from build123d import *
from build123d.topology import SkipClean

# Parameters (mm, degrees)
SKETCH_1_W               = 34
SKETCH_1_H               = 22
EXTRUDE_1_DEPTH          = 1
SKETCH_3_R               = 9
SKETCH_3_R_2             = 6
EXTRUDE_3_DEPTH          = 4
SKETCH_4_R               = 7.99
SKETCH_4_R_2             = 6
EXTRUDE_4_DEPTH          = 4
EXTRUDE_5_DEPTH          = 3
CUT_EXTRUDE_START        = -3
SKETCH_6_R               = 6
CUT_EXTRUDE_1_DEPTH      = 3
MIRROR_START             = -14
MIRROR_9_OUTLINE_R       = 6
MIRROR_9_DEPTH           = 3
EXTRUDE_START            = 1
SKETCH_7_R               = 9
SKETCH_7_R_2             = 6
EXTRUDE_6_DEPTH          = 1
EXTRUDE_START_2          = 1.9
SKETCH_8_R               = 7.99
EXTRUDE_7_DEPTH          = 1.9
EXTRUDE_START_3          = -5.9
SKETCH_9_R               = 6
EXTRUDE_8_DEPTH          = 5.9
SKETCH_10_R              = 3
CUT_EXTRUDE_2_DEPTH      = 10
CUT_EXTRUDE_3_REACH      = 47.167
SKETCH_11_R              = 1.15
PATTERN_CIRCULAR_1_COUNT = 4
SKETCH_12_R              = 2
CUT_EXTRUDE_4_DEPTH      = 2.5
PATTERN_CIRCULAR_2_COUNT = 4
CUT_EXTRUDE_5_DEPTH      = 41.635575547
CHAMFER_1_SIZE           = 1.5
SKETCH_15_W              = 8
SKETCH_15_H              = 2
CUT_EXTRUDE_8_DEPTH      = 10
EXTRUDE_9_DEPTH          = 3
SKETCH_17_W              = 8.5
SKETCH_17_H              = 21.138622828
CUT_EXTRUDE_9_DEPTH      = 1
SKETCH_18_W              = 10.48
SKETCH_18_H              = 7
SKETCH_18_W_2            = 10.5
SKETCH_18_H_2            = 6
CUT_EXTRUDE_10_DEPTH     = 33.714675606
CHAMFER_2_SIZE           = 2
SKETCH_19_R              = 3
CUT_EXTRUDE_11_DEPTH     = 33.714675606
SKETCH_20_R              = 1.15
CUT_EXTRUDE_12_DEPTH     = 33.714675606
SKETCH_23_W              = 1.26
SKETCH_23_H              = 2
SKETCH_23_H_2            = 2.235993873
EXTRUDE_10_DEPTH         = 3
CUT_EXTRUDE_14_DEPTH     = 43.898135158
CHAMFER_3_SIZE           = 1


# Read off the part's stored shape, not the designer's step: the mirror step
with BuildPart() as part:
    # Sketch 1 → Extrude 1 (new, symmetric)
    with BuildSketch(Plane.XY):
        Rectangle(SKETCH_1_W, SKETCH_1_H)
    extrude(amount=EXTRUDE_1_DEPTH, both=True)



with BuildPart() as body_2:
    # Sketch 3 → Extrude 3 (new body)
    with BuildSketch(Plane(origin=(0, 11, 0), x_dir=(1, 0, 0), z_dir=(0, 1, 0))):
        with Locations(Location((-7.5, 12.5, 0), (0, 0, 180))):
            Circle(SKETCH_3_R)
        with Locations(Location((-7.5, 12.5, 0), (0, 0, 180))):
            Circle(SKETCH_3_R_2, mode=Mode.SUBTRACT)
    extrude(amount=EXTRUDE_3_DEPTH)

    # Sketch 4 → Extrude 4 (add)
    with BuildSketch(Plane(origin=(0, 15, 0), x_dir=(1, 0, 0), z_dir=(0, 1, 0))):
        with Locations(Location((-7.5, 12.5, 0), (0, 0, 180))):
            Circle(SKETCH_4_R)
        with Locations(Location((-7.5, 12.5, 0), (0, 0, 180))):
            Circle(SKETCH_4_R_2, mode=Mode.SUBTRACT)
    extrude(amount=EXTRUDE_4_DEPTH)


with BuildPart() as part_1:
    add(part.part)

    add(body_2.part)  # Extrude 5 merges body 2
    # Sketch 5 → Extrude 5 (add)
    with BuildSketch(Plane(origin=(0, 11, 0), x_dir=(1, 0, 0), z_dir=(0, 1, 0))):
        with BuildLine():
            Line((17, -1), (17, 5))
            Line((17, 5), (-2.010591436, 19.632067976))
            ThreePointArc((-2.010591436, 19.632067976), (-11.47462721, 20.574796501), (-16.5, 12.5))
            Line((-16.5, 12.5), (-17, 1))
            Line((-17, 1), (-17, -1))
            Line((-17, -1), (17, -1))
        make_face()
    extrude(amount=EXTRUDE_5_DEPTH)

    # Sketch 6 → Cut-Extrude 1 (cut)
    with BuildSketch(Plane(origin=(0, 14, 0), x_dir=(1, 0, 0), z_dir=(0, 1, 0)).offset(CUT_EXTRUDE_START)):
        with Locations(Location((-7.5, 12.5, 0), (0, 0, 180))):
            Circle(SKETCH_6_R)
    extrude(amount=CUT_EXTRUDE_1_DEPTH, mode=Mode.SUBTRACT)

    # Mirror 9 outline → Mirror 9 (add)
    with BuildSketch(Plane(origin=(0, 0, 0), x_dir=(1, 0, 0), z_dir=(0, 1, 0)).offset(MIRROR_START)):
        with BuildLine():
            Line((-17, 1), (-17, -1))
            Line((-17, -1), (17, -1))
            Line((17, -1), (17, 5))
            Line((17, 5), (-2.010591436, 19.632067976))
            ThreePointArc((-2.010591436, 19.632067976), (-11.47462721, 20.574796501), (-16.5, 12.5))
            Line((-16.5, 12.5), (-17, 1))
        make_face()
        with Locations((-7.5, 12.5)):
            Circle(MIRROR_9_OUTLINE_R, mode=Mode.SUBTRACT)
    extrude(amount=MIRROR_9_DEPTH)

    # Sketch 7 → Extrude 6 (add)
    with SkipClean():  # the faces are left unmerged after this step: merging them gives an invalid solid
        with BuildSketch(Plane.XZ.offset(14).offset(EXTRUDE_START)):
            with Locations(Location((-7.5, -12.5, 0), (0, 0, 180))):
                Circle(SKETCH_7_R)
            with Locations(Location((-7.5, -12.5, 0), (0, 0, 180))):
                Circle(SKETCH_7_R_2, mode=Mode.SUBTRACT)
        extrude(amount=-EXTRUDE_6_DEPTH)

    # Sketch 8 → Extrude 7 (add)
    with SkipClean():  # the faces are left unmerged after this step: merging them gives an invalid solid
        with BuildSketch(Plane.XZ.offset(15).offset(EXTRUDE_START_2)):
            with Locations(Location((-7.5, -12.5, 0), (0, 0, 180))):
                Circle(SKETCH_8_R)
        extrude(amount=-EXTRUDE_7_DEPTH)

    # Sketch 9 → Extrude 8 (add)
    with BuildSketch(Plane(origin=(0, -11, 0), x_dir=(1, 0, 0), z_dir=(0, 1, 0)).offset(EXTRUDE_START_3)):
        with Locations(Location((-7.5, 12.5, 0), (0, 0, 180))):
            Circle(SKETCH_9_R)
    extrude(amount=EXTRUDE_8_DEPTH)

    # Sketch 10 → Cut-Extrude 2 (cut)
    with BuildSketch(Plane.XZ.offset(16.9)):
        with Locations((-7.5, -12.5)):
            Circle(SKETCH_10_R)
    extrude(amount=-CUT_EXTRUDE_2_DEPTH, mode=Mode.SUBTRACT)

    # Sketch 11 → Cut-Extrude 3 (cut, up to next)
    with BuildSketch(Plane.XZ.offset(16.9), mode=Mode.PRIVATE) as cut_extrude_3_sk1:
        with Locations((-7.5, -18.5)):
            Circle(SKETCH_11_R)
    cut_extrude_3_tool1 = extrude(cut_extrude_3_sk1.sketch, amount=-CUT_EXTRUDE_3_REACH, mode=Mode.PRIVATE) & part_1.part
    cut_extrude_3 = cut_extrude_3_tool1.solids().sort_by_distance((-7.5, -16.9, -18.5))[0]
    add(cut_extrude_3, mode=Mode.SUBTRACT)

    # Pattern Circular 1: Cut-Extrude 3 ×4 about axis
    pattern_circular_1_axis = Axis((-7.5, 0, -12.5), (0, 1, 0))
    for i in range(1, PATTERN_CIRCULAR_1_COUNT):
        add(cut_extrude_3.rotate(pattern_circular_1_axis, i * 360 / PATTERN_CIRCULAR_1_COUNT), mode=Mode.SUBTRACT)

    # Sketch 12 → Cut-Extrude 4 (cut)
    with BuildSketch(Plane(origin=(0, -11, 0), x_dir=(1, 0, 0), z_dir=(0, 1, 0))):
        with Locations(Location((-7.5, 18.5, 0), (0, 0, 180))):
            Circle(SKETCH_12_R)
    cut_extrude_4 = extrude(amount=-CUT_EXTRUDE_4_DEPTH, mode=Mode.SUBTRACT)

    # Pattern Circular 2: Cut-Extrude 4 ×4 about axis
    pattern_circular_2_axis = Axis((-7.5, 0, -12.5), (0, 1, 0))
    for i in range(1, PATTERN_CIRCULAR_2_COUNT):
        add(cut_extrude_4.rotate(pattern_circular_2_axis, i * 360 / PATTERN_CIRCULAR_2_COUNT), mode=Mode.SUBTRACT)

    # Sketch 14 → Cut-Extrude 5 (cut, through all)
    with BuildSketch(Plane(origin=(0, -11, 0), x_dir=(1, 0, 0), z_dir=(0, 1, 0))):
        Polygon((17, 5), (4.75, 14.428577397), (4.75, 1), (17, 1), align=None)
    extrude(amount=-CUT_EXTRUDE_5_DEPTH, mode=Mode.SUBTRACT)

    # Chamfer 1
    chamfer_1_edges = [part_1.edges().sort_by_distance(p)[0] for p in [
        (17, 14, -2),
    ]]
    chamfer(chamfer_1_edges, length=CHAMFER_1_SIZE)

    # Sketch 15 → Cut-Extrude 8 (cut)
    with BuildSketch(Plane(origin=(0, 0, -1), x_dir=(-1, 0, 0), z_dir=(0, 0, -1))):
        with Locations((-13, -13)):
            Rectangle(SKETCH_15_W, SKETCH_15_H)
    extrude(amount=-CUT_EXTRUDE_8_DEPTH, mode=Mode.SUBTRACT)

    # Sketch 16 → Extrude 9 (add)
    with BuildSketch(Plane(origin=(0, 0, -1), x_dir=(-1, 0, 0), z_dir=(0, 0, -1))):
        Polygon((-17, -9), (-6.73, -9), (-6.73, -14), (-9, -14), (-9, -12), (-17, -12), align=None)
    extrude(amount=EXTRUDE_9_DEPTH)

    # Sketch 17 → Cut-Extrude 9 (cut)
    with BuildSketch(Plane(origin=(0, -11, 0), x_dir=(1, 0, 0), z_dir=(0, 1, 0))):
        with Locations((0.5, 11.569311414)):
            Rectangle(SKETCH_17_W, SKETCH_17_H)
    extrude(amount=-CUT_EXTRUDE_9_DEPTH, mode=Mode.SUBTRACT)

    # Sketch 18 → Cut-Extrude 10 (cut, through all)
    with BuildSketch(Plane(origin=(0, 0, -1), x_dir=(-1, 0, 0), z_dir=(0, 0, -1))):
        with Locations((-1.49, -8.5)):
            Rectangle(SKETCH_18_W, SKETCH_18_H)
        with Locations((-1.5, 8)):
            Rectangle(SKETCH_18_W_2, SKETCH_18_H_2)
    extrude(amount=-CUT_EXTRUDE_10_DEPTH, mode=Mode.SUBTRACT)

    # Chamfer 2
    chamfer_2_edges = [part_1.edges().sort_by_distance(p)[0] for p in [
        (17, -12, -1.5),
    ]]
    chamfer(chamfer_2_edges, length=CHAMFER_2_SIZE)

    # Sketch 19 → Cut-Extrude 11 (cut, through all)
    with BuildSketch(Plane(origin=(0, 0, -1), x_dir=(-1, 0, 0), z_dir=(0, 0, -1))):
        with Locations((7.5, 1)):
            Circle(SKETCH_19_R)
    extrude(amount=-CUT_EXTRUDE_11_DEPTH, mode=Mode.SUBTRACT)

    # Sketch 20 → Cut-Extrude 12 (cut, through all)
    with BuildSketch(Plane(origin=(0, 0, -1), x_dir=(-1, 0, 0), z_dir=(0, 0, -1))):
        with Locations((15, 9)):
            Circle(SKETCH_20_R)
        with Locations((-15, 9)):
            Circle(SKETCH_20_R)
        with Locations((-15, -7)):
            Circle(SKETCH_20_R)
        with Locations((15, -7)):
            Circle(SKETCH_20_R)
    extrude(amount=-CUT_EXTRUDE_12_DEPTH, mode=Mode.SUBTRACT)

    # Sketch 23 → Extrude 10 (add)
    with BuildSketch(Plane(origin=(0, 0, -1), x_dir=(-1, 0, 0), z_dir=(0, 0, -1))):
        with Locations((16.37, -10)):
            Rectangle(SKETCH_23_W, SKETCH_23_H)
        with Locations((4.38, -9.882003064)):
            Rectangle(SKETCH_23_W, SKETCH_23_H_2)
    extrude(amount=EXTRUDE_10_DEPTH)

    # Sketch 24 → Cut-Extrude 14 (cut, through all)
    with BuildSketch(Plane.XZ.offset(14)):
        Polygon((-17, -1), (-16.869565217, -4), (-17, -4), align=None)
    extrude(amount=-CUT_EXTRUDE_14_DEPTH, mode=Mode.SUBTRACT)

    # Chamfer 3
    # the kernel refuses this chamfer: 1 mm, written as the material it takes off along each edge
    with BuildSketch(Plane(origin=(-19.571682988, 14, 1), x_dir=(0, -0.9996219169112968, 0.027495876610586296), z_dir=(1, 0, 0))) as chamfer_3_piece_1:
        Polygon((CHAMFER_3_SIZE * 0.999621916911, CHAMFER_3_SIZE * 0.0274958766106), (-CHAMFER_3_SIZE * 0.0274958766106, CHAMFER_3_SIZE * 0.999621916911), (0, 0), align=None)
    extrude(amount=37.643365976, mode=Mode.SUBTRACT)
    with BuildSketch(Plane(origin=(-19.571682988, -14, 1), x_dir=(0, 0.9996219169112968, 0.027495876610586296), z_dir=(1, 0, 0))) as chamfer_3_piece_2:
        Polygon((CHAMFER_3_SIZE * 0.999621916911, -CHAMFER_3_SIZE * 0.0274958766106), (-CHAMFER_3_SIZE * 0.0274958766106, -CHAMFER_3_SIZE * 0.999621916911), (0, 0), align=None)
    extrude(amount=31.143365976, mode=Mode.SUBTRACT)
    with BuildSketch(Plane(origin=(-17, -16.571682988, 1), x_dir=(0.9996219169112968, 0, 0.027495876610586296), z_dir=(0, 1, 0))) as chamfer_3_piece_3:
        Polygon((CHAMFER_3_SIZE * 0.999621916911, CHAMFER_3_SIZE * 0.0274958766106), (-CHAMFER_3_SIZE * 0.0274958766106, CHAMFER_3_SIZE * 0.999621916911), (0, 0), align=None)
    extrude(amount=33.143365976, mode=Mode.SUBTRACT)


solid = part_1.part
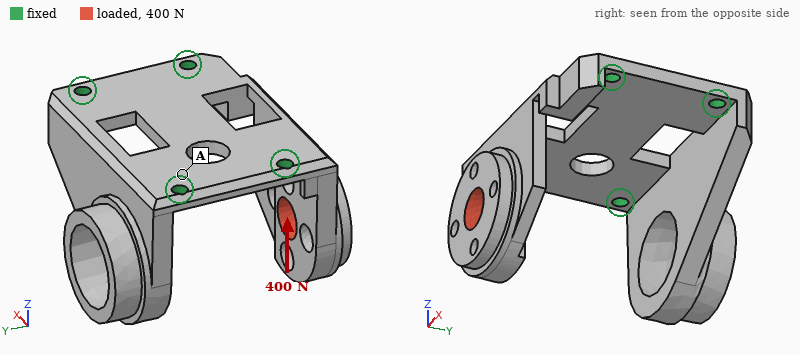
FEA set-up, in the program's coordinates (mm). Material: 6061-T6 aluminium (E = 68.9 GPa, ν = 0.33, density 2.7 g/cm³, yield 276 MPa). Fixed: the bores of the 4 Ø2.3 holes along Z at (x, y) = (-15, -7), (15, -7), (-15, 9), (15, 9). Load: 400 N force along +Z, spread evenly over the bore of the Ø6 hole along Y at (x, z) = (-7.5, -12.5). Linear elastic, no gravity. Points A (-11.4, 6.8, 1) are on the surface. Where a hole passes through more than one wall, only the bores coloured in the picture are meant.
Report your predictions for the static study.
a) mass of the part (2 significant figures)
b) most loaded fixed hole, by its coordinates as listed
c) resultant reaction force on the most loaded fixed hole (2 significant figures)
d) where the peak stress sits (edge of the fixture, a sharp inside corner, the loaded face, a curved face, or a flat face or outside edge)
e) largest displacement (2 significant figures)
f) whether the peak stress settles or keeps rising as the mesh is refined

12 g
(-15, -7)
320 N
edge of the fixture
0.27 mm
keeps rising
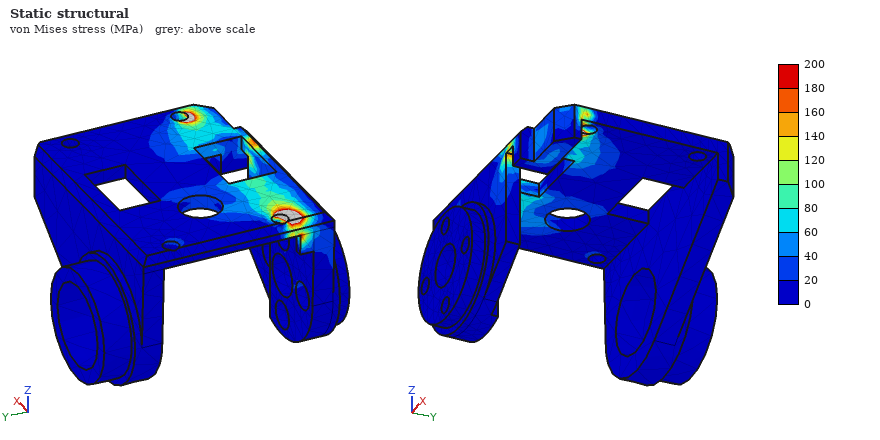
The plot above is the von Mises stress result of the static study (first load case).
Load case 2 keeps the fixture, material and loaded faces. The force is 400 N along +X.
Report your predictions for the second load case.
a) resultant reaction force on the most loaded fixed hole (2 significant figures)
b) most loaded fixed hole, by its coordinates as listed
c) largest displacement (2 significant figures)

370 N
(-15, -7)
0.15 mm
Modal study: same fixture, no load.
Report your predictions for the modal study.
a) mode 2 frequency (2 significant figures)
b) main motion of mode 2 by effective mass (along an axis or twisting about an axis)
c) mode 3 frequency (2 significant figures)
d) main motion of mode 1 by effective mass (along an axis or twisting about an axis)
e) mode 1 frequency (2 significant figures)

3200 Hz
along Y
5000 Hz
along Y
2400 Hz
